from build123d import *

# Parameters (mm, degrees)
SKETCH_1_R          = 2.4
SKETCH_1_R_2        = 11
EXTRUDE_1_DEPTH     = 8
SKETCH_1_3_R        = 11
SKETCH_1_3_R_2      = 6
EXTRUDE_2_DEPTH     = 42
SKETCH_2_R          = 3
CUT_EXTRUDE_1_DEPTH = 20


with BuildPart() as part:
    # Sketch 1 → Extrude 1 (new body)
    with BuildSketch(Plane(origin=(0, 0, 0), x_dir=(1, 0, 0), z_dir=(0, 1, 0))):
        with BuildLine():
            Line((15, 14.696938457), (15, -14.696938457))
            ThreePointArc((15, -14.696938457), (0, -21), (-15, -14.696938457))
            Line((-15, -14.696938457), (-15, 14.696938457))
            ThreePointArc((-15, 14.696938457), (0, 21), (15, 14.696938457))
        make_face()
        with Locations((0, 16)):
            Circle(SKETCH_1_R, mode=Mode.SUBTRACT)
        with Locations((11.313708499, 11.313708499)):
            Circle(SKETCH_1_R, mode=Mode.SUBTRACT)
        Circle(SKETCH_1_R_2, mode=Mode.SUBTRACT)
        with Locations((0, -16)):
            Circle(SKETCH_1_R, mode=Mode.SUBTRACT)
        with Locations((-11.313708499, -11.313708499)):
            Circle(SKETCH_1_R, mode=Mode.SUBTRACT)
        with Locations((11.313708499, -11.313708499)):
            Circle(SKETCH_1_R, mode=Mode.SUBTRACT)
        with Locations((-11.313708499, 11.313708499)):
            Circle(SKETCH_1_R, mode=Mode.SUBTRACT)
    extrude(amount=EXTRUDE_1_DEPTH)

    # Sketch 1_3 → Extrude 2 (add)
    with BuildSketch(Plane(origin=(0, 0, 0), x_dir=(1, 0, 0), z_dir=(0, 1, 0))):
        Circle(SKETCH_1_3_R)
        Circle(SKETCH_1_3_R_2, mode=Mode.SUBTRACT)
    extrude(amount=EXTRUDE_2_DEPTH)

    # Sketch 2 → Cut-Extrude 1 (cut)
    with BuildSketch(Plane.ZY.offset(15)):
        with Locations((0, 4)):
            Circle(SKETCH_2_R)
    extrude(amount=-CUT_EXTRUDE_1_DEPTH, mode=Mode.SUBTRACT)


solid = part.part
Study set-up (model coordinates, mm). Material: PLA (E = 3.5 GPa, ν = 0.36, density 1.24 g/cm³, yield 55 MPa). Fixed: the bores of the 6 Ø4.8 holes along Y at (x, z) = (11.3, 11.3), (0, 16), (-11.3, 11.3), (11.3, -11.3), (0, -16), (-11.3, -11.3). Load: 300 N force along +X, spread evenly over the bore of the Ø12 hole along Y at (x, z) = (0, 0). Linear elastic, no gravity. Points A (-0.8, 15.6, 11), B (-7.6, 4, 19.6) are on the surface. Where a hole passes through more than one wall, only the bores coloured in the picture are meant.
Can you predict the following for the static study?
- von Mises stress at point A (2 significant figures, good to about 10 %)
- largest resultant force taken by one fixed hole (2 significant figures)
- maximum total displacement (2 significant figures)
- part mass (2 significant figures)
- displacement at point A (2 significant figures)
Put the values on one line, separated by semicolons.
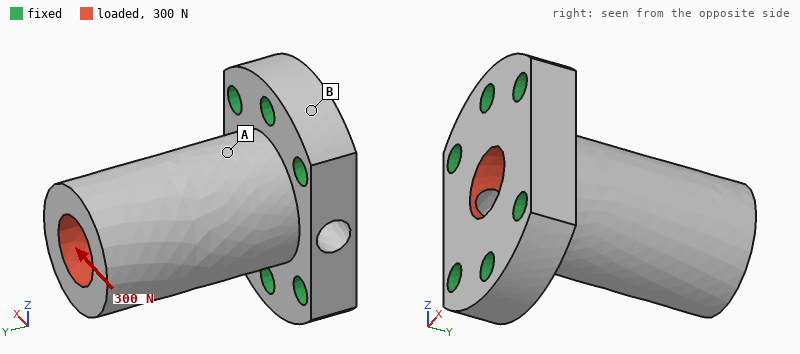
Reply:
1.6 MPa; 140 N; 95 µm; 20 g; 20 µm
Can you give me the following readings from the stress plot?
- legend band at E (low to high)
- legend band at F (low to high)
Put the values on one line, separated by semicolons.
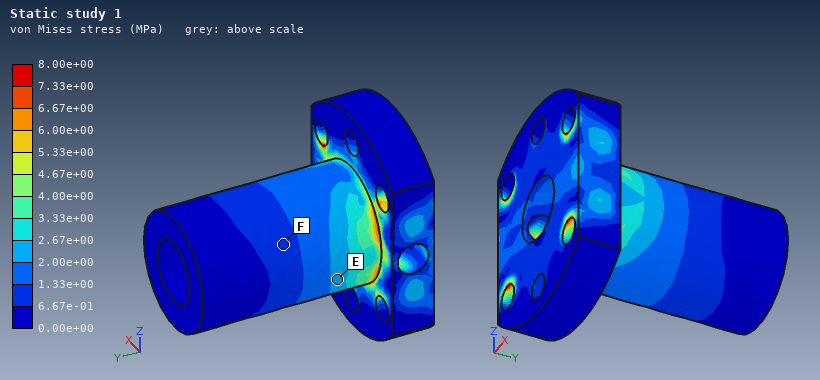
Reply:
2.00e+00 to 2.67e+00 MPa; 6.67e-01 to 1.33e+00 MPa
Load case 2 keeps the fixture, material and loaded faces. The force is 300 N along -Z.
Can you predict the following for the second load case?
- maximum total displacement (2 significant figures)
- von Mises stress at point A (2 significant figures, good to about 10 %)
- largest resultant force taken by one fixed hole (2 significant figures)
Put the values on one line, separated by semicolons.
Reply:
79 µm; 2.5 MPa; 120 N
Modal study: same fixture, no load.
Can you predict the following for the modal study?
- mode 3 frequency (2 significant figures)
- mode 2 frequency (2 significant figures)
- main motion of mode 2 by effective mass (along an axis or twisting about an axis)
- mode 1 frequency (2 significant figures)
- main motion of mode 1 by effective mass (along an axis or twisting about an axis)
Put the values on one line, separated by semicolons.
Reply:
6900 Hz; 3200 Hz; along Z; 2900 Hz; along X
